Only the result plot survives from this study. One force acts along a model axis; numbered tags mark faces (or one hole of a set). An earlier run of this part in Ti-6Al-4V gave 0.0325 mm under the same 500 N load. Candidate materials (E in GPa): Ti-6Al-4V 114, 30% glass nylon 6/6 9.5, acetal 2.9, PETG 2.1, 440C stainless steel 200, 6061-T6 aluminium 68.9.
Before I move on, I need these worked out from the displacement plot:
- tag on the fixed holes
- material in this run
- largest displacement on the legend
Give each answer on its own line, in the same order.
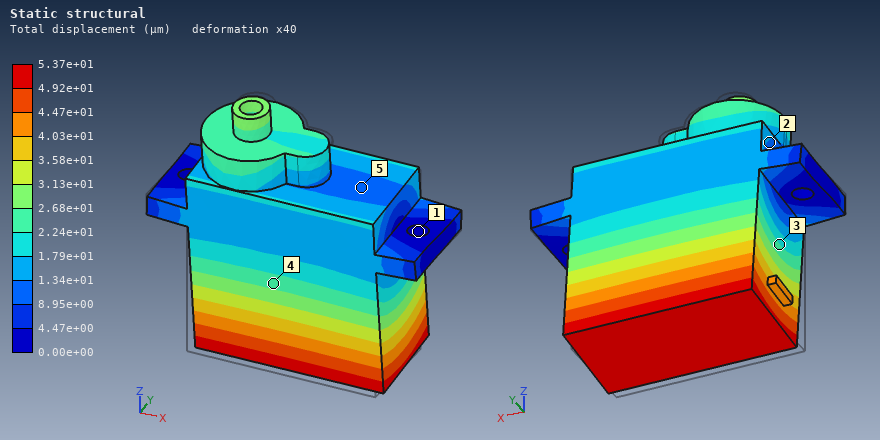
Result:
1
6061-T6 aluminium
5.37e+01 µm
